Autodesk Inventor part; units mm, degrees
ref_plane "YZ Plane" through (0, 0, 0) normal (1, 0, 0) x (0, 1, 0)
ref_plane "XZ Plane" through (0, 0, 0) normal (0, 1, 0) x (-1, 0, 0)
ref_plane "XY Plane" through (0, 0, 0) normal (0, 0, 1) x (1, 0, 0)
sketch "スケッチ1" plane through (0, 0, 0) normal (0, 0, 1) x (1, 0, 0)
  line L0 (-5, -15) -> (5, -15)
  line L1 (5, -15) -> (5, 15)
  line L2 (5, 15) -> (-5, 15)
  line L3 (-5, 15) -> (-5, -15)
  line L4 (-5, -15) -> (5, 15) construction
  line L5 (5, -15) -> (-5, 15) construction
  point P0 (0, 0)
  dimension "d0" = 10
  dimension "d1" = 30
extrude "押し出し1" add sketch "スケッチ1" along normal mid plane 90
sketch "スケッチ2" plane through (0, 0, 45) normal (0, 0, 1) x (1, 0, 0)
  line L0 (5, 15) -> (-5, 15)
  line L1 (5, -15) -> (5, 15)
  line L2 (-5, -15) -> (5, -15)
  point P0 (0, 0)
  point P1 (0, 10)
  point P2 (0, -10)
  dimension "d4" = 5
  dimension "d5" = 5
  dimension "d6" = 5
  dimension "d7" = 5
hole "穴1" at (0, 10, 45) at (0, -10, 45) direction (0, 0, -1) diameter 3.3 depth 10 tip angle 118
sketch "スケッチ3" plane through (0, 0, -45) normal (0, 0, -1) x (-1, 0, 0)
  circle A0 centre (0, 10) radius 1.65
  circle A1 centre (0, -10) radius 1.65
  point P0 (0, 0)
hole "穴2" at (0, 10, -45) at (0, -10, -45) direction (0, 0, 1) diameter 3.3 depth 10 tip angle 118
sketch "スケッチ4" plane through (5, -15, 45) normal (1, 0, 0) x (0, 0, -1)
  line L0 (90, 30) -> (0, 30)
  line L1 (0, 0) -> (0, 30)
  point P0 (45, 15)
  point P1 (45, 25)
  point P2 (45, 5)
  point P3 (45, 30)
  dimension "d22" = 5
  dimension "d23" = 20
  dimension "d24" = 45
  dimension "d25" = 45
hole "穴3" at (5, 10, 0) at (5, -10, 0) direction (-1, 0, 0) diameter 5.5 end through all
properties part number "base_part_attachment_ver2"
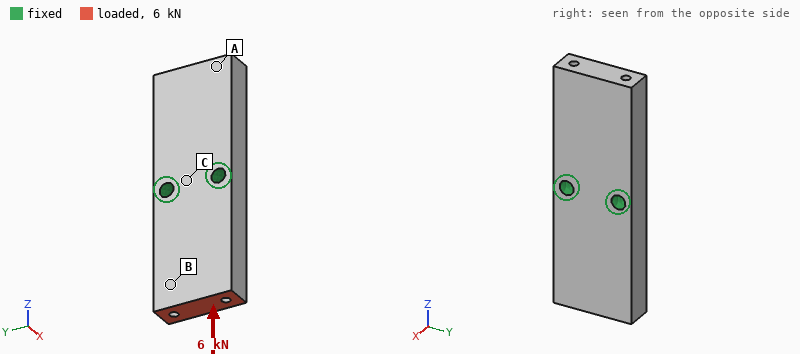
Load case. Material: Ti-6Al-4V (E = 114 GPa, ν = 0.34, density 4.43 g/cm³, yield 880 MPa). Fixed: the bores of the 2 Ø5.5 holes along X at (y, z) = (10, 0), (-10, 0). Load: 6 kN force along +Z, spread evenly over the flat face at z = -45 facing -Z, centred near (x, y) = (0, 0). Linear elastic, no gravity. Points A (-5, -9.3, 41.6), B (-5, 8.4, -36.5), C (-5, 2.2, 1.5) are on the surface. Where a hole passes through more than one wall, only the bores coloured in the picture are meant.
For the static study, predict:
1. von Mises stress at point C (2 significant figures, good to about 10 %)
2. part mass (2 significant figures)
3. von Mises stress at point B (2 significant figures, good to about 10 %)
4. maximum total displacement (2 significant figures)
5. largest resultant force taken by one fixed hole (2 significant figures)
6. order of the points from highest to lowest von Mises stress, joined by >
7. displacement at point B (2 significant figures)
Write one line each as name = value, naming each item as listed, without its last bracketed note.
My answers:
von Mises stress at point C = 7.6 MPa
part mass = 120 g
von Mises stress at point B = 21 MPa
maximum total displacement = 8.0 µm
largest resultant force taken by one fixed hole = 3.0 kN
order of the points from highest to lowest von Mises stress, joined by > = B > C > A
displacement at point B = 6.4 µm
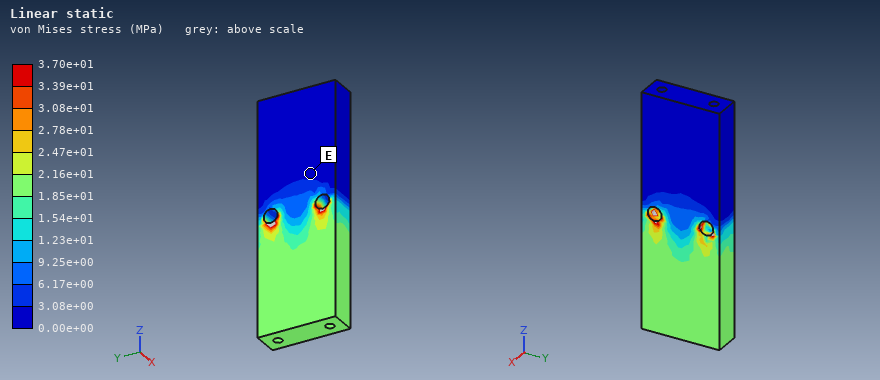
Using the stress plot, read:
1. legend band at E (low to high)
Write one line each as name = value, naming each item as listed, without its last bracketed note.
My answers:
legend band at E = 0.00e+00 to 3.08e+00 MPa
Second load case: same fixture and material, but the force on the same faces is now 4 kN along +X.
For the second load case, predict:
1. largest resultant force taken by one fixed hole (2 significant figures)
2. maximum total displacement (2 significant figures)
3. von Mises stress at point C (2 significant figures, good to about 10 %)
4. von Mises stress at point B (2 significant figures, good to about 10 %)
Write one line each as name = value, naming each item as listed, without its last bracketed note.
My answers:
largest resultant force taken by one fixed hole = 2.0 kN
maximum total displacement = 0.43 mm
von Mises stress at point C = 110 MPa
von Mises stress at point B = 71 MPa
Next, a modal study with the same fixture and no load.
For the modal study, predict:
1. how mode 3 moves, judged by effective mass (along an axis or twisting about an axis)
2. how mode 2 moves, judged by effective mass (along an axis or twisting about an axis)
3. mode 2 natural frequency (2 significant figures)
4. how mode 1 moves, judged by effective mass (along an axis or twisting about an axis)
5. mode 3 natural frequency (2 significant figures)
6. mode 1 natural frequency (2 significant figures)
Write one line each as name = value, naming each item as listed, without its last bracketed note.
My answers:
how mode 3 moves, judged by effective mass = twisting about X
how mode 2 moves, judged by effective mass = along X
mode 2 natural frequency = 4300 Hz
how mode 1 moves, judged by effective mass = twisting about Y
mode 3 natural frequency = 9900 Hz
mode 1 natural frequency = 4000 Hz
